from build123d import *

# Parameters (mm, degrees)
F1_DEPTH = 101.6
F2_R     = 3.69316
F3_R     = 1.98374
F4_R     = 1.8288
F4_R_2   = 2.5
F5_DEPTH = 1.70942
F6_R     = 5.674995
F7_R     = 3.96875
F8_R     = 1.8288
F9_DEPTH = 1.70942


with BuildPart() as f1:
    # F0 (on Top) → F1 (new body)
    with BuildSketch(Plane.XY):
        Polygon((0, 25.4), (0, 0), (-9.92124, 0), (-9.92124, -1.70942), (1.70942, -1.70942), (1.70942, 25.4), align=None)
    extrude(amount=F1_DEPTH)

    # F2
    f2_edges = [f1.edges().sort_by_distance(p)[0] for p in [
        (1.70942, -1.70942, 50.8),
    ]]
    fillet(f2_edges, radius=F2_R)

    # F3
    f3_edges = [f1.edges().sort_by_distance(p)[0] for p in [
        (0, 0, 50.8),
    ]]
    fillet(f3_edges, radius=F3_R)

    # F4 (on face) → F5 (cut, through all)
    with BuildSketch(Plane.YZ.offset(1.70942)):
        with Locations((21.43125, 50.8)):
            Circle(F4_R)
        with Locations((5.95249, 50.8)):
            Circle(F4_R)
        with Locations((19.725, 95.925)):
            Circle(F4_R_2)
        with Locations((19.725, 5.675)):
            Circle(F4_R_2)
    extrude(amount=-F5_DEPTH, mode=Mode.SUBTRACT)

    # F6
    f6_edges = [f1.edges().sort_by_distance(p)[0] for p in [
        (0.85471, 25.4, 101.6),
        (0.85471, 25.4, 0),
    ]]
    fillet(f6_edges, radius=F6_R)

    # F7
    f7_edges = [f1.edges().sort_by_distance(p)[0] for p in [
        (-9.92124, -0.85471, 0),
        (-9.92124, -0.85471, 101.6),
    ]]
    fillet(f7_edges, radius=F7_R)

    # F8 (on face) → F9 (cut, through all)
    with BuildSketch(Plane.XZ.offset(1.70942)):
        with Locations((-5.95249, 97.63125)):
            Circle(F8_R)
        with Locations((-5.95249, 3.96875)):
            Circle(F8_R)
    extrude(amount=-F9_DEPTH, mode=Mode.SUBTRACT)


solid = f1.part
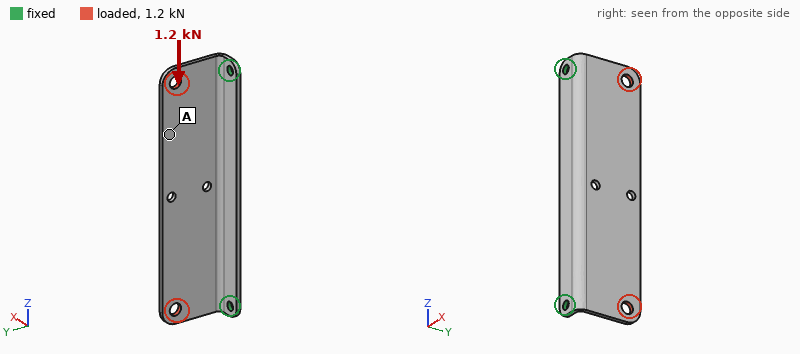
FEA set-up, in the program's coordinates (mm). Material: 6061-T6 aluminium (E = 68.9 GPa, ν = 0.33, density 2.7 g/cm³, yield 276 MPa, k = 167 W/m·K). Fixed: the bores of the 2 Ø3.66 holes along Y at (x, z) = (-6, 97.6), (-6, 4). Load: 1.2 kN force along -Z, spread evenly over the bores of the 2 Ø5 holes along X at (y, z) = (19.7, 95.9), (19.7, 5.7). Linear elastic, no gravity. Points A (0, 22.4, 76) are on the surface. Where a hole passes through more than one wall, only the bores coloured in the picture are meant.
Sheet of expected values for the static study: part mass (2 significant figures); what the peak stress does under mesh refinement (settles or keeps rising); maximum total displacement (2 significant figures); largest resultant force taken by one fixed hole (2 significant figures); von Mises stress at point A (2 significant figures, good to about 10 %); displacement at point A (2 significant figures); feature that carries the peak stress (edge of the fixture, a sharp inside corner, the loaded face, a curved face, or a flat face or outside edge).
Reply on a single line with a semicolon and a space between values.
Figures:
16 g; keeps rising; 0.18 mm; 660 N; 23 MPa; 0.094 mm; edge of the fixture
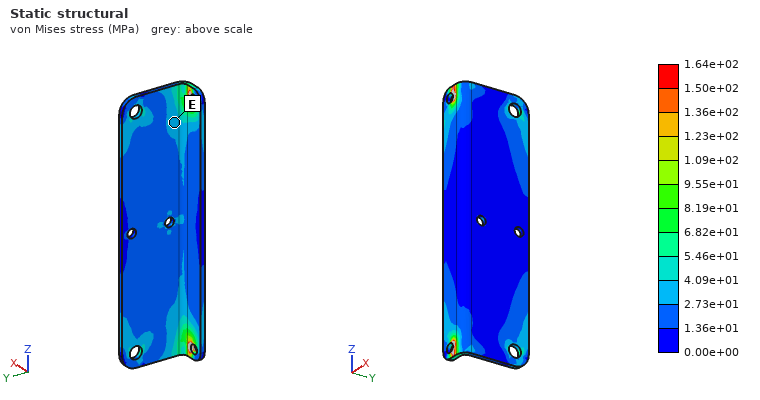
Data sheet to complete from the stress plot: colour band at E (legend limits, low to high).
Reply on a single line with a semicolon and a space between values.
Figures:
2.73e+01 to 4.09e+01 MPa
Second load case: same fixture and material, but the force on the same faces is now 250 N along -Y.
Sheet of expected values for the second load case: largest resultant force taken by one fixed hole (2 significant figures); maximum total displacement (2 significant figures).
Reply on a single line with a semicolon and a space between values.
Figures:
130 N; 0.13 mm
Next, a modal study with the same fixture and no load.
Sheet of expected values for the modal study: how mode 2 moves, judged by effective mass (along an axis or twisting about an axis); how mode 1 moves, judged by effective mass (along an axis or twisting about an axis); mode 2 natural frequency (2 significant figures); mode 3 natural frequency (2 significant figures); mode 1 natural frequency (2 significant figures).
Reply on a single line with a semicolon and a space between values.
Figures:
twisting about Y; along X; 1800 Hz; 2700 Hz; 910 Hz
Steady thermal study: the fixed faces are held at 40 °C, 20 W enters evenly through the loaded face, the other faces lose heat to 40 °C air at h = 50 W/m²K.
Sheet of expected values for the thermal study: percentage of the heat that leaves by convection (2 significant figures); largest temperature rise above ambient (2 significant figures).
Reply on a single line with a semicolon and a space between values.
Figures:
34 %; 47 K
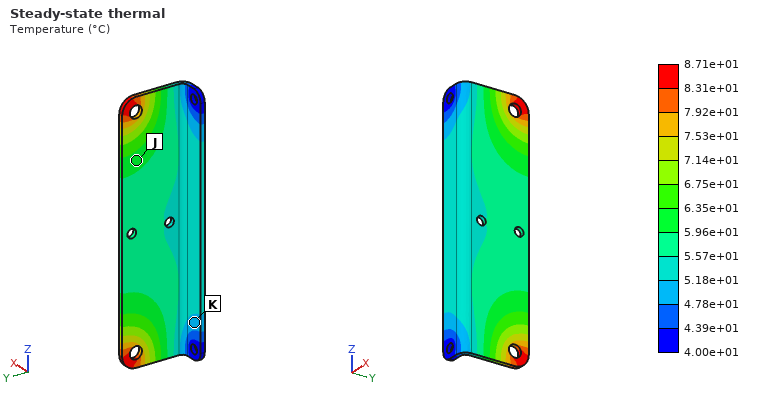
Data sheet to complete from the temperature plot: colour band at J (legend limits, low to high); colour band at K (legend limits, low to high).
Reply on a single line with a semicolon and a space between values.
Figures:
5.96e+01 to 6.35e+01 °C; 4.78e+01 to 5.18e+01 °C
